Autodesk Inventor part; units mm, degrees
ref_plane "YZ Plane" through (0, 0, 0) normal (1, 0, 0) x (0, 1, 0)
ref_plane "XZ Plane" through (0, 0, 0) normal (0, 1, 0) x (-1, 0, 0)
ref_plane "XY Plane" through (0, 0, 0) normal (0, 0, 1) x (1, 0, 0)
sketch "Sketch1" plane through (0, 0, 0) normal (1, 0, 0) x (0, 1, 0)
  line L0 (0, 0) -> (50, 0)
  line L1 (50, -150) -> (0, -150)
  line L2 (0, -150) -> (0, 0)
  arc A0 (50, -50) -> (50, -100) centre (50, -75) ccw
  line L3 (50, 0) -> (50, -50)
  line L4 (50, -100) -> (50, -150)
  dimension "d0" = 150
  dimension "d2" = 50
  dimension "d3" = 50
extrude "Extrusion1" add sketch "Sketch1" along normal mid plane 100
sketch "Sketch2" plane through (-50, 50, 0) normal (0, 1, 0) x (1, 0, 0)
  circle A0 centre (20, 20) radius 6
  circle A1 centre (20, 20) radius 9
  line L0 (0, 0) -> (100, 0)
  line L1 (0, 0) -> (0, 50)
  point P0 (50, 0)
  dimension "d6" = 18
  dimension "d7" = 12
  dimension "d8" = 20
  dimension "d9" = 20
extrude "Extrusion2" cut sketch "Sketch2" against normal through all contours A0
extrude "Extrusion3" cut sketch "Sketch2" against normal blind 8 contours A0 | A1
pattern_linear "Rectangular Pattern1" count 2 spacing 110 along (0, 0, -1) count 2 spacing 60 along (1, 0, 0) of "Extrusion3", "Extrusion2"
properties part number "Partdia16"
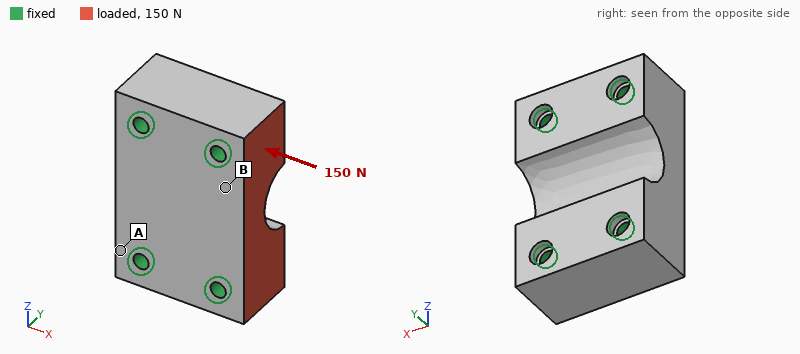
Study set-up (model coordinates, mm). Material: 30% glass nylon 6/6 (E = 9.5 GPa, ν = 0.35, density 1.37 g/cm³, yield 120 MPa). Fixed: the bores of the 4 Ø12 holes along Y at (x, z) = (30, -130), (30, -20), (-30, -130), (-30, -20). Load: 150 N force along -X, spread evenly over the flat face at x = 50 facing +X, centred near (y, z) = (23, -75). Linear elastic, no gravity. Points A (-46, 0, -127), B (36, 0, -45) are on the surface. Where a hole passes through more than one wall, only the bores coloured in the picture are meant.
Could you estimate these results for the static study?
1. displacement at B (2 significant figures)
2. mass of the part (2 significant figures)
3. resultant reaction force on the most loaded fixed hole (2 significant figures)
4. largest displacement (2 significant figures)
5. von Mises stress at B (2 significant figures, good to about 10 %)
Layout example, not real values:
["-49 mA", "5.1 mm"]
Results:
["0.12 µm", "860 g", "56 N", "0.21 µm", "0.021 MPa"]
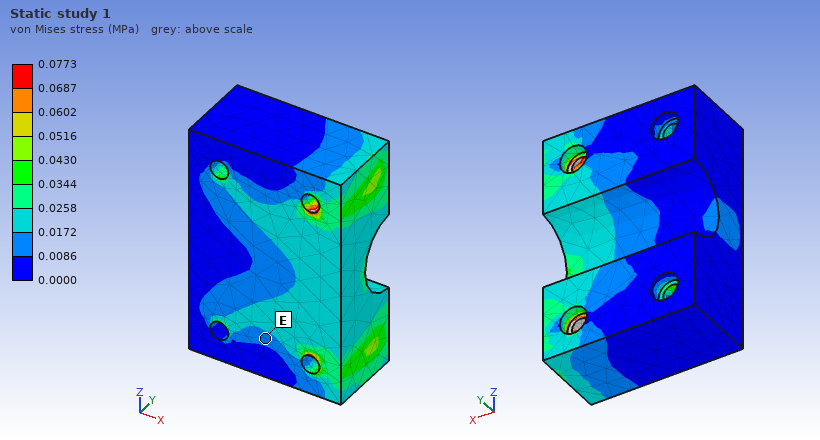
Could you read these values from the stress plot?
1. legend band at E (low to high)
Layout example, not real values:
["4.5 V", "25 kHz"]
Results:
["0.0086 to 0.0172 MPa"]
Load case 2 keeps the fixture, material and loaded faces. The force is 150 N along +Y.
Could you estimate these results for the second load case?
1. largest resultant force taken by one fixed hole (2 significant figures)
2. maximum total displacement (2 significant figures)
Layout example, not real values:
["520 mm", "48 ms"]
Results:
["80 N", "0.79 µm"]
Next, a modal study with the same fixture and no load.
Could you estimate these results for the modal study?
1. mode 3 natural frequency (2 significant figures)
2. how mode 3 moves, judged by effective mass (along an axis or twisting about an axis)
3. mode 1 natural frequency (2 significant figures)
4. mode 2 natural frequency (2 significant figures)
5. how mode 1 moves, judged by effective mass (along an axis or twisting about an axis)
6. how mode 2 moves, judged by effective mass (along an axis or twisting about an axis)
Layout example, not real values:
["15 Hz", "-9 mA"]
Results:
["7600 Hz", "along X", "5300 Hz", "6400 Hz", "along Y", "along X"]
